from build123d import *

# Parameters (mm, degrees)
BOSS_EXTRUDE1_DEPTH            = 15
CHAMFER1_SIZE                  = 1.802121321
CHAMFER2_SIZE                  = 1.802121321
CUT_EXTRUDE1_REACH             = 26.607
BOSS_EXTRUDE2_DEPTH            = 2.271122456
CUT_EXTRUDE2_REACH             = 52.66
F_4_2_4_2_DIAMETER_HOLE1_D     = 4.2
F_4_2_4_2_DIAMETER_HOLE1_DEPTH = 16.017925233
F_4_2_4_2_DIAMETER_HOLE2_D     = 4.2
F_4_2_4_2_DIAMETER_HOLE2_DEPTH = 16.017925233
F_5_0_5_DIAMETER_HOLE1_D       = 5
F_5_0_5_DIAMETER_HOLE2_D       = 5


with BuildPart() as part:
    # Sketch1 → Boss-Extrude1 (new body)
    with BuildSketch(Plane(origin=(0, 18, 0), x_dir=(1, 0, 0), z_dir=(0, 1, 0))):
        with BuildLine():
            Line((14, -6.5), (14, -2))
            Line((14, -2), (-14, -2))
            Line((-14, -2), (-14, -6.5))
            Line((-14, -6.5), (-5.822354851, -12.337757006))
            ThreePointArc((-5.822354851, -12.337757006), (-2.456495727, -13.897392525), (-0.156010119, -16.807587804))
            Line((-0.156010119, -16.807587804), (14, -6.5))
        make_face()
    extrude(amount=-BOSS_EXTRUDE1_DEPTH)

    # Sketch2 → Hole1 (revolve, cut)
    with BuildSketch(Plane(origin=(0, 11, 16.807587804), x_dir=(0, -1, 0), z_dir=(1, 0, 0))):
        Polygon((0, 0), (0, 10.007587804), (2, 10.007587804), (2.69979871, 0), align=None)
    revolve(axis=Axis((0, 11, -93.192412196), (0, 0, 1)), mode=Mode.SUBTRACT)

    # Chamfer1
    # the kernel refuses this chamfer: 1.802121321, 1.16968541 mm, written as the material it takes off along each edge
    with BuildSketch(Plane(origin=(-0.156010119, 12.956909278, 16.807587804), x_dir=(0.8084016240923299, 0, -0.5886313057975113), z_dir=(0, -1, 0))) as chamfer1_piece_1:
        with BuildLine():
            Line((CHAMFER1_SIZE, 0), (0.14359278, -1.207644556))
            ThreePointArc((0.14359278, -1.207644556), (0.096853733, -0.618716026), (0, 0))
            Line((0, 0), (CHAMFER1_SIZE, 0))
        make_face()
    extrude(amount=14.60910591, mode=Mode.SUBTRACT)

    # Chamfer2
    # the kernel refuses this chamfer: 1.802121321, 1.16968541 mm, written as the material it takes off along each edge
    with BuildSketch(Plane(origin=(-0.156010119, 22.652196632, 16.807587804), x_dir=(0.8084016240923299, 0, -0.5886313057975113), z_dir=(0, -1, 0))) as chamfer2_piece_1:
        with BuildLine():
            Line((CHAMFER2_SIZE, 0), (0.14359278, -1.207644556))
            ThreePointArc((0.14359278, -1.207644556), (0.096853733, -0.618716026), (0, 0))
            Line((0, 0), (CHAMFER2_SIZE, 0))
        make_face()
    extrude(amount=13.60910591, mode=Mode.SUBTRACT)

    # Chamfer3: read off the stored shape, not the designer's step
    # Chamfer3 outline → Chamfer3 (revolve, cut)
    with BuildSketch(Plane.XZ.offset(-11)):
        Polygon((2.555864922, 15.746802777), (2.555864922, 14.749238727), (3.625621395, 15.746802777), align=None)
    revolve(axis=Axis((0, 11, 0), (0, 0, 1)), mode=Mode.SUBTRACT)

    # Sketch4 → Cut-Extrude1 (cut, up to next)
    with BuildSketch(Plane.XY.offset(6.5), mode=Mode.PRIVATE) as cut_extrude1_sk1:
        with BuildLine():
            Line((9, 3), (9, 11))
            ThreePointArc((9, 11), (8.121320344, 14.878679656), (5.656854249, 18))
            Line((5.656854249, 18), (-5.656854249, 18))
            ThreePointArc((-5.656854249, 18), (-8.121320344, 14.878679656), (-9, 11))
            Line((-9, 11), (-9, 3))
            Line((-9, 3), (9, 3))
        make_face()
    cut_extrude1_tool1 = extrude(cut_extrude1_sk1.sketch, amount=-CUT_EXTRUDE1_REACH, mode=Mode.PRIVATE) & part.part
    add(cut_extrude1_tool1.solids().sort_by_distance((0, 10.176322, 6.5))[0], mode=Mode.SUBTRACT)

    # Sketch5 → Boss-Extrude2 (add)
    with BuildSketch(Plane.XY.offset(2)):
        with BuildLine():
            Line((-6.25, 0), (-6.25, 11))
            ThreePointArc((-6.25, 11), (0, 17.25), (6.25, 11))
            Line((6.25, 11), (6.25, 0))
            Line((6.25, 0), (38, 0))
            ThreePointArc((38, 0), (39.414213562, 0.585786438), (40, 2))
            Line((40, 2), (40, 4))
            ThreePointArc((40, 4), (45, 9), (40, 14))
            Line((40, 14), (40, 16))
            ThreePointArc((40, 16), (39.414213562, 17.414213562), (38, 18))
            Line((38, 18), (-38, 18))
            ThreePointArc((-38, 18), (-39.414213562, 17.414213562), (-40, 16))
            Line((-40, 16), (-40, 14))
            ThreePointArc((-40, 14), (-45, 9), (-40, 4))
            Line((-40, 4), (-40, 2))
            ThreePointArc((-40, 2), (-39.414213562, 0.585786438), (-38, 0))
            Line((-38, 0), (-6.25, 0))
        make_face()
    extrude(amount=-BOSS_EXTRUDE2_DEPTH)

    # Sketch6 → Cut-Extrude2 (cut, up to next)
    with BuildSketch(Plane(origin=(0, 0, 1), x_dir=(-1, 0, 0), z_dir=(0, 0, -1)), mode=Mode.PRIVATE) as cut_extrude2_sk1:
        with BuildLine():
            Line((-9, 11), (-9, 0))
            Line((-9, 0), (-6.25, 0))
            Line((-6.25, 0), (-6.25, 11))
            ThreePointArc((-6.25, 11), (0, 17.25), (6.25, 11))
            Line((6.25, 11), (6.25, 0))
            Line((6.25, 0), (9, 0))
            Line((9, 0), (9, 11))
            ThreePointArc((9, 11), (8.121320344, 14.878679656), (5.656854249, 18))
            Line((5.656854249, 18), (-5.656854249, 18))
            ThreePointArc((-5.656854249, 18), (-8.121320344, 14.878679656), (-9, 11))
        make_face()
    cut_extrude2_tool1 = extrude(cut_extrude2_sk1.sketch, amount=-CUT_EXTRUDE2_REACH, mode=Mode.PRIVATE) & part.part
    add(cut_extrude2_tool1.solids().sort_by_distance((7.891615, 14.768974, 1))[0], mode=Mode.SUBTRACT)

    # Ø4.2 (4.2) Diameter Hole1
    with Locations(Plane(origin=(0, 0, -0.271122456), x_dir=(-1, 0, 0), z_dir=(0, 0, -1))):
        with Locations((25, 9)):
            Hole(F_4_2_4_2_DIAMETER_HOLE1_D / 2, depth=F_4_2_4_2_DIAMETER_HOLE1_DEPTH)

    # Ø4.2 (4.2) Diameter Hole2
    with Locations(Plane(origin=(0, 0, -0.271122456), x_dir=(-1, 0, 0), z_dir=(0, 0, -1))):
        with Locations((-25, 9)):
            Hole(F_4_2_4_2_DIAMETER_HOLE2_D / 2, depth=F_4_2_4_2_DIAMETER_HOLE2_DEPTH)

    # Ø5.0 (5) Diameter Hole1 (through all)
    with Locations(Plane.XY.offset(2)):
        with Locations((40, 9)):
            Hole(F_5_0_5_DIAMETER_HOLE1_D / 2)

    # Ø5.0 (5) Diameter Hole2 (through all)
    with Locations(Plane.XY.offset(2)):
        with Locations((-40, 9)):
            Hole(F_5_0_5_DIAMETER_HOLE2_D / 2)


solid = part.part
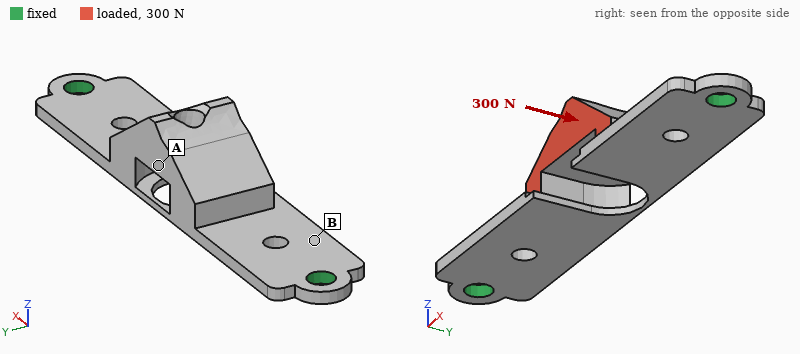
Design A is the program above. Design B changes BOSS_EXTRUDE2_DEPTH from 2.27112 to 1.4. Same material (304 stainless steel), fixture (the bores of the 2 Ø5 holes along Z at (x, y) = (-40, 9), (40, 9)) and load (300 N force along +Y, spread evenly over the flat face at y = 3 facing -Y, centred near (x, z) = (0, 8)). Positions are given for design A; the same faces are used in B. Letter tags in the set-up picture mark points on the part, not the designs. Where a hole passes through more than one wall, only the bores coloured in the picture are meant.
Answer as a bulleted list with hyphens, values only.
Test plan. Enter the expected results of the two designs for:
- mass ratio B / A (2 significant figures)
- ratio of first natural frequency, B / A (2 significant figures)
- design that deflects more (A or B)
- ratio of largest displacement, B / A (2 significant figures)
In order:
- 0.80
- 0.55
- B
- 3.3
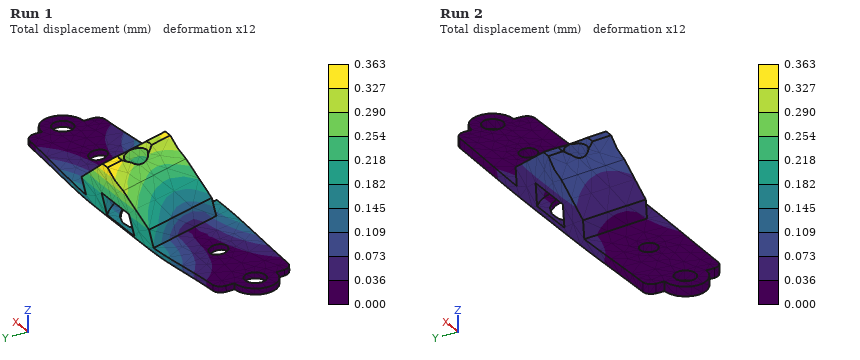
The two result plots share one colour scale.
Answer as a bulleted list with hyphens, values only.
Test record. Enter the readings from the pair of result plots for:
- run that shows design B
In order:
- Run 1
